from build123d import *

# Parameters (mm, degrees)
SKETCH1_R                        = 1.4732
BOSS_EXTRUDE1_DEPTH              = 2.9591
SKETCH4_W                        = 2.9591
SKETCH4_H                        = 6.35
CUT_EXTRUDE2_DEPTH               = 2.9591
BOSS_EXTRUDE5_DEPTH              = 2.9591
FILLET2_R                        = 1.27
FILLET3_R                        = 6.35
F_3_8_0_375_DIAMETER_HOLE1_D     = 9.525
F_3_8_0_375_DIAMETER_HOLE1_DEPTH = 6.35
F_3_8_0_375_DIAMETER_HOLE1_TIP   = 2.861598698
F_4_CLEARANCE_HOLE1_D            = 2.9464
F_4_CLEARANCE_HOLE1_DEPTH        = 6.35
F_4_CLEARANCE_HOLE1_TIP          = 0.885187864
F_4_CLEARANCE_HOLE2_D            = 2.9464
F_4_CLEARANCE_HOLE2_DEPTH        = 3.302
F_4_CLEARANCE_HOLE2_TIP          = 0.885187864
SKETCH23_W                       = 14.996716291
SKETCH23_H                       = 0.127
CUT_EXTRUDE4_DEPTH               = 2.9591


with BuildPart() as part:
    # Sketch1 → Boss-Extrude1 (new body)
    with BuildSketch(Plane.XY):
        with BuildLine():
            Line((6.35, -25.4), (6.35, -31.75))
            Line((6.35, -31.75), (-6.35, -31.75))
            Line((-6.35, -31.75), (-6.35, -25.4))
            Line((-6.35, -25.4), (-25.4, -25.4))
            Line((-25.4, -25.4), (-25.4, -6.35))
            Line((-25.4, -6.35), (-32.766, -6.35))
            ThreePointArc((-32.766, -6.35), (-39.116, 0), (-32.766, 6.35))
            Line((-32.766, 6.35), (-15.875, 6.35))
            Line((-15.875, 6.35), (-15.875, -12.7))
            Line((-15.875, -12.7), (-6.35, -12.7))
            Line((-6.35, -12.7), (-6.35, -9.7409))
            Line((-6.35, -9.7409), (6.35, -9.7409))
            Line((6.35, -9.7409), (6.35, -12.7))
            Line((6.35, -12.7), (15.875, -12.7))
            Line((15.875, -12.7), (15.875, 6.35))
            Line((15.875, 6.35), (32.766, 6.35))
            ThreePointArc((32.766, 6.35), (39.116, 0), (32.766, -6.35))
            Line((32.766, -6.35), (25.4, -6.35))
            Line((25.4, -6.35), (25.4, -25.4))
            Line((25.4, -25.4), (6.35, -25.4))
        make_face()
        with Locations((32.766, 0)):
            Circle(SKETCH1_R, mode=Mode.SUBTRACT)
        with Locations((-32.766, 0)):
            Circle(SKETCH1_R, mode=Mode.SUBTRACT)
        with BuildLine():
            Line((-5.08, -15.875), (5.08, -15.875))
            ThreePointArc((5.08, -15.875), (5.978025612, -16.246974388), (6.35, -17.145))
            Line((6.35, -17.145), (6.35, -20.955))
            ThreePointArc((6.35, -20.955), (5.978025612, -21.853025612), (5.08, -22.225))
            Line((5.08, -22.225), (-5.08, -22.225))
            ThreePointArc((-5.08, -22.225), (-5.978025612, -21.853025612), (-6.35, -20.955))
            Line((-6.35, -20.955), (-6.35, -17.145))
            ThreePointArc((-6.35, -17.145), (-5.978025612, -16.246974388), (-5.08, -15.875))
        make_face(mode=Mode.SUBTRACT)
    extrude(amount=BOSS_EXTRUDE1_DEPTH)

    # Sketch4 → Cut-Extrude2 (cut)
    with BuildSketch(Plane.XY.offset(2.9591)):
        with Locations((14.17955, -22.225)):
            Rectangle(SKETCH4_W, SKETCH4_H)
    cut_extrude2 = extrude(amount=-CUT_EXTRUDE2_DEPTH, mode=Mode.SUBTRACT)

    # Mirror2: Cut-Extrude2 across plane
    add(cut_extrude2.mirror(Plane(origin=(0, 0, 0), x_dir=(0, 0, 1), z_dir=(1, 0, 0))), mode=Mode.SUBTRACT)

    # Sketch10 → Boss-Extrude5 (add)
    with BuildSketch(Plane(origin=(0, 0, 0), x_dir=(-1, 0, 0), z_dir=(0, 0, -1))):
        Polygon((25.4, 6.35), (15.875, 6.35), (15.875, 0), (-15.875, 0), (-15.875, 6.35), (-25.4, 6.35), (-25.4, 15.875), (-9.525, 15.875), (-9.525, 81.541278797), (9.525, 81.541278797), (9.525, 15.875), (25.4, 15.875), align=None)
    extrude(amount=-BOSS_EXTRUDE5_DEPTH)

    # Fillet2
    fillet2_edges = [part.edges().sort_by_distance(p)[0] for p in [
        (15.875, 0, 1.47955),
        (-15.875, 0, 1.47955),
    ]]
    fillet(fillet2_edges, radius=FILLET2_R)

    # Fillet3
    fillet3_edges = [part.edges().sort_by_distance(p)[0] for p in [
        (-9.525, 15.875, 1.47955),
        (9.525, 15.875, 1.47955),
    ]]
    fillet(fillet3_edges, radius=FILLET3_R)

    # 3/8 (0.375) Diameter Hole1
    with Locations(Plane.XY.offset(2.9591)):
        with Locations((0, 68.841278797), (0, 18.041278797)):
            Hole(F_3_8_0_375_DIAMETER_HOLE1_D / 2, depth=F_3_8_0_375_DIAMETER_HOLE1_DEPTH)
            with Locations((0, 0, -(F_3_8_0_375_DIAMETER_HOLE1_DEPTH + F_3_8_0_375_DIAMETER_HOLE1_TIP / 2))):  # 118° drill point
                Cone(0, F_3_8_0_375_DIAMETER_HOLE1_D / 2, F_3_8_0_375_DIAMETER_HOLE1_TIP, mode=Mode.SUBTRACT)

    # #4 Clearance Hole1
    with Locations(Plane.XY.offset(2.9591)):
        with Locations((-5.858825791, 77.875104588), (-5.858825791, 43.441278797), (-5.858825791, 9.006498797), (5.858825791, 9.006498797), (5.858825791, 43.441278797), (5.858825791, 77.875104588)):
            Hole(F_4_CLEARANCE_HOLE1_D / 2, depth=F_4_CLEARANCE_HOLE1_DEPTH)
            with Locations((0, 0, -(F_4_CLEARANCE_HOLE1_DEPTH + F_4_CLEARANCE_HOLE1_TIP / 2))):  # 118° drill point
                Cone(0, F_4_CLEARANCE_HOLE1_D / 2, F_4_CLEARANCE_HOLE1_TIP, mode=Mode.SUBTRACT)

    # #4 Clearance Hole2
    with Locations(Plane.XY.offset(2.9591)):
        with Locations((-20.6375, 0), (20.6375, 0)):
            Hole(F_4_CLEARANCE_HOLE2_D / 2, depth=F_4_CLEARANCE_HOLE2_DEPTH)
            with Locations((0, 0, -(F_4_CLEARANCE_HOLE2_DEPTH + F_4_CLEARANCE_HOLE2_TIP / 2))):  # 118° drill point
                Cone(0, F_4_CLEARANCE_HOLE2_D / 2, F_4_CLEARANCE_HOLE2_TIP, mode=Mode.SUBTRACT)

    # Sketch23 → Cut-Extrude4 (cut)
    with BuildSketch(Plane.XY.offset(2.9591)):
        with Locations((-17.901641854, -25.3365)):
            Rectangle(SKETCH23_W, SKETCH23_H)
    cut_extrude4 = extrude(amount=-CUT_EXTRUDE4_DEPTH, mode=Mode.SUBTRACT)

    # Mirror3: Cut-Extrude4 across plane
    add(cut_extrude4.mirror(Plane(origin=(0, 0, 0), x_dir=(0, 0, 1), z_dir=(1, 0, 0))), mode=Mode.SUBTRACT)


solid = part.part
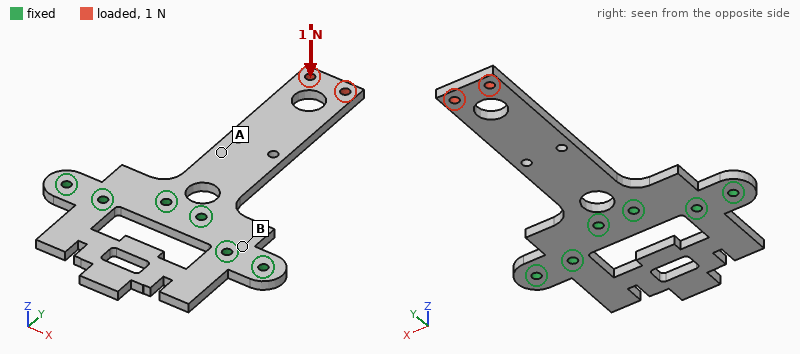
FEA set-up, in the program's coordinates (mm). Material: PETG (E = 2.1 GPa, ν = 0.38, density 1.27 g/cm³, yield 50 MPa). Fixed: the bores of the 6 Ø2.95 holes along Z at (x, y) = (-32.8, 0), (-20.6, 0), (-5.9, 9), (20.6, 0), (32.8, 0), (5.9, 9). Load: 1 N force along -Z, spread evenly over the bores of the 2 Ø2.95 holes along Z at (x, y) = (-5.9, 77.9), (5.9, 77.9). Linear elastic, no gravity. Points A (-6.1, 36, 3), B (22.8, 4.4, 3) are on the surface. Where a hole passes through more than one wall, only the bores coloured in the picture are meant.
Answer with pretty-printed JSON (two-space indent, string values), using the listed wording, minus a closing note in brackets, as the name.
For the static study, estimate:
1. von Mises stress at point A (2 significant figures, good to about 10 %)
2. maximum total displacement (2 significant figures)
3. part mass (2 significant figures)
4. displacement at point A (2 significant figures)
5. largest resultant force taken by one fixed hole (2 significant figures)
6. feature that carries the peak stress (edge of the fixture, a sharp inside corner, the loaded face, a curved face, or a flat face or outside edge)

{
  "von Mises stress at point A": "1.5 MPa",
  "maximum total displacement": "1.5 mm",
  "part mass": "12 g",
  "displacement at point A": "0.28 mm",
  "largest resultant force taken by one fixed hole": "1.3 N",
  "feature that carries the peak stress": "a curved face"
}
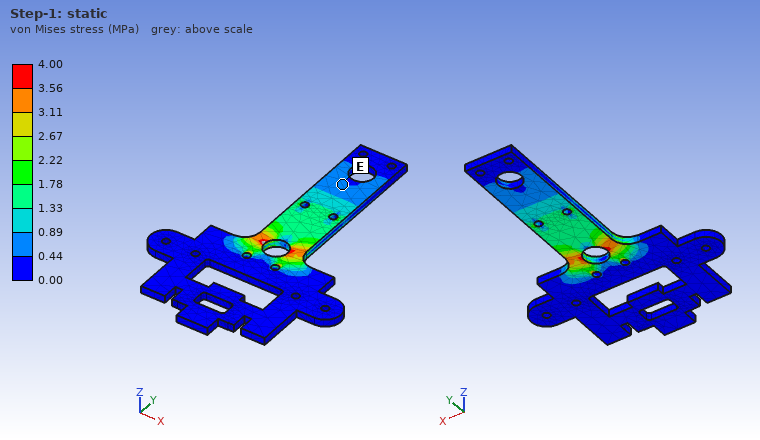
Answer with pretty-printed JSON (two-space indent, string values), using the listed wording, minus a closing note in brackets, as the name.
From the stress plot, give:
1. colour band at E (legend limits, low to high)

{
  "colour band at E": "0.44 to 0.89 MPa"
}
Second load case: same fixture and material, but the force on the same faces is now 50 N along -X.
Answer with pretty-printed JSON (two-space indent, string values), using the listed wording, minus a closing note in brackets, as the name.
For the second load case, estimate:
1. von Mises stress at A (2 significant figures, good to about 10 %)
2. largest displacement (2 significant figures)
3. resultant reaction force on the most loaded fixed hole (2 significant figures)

{
  "von Mises stress at A": "7.2 MPa",
  "largest displacement": "1.6 mm",
  "resultant reaction force on the most loaded fixed hole": "130 N"
}
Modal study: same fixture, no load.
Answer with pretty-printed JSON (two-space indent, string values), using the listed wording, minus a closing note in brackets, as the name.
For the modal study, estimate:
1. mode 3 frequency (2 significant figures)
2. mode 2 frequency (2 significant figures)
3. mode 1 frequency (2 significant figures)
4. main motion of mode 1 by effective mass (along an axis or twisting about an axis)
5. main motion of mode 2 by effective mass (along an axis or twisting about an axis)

{
  "mode 3 frequency": "740 Hz",
  "mode 2 frequency": "550 Hz",
  "mode 1 frequency": "120 Hz",
  "main motion of mode 1 by effective mass": "along Z",
  "main motion of mode 2 by effective mass": "along Z"
}
